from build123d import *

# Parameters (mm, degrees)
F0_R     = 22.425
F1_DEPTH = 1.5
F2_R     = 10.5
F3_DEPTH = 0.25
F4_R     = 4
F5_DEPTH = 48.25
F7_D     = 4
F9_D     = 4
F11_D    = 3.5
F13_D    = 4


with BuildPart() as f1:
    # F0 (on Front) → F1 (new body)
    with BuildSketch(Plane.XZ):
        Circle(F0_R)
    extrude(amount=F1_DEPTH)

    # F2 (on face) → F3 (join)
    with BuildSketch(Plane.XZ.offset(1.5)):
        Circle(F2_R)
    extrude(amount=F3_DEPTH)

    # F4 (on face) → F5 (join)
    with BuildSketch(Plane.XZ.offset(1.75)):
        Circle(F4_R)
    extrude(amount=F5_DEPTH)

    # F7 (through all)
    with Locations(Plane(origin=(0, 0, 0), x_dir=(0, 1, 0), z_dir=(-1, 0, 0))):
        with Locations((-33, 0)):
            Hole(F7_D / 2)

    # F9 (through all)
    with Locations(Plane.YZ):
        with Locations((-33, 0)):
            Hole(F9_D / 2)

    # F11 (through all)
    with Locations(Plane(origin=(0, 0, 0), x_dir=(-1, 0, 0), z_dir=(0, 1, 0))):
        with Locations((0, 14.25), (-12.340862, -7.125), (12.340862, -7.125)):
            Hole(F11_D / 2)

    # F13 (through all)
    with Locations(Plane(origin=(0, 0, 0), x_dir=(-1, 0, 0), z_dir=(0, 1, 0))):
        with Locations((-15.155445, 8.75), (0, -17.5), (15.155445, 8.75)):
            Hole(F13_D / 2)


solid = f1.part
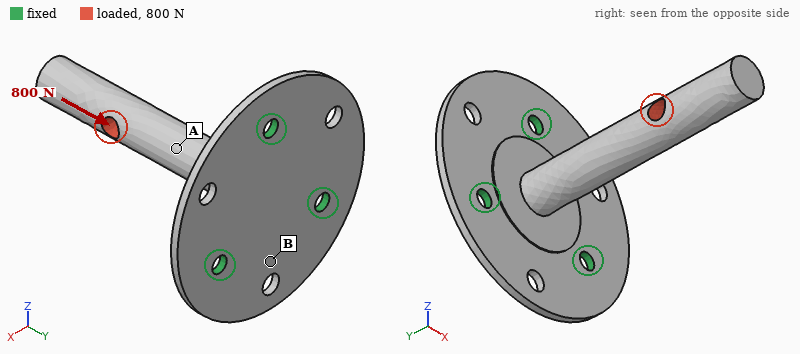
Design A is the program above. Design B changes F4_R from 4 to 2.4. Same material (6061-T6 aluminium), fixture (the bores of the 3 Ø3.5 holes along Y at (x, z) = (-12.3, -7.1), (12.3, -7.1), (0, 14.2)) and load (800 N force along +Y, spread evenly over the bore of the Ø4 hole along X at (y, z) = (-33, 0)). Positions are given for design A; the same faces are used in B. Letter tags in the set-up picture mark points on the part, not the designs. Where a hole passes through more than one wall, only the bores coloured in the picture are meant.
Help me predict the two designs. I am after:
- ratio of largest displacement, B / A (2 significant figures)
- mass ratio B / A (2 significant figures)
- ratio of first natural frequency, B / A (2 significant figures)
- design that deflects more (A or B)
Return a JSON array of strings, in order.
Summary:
["1.7", "0.68", "0.80", "B"]
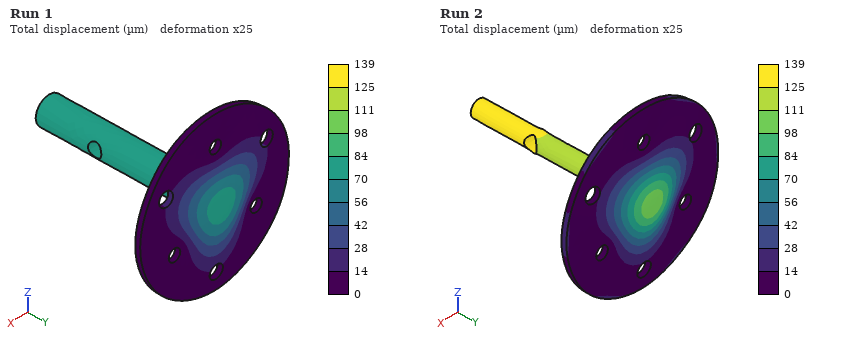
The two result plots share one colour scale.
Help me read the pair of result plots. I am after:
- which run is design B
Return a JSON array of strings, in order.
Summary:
["Run 2"]
